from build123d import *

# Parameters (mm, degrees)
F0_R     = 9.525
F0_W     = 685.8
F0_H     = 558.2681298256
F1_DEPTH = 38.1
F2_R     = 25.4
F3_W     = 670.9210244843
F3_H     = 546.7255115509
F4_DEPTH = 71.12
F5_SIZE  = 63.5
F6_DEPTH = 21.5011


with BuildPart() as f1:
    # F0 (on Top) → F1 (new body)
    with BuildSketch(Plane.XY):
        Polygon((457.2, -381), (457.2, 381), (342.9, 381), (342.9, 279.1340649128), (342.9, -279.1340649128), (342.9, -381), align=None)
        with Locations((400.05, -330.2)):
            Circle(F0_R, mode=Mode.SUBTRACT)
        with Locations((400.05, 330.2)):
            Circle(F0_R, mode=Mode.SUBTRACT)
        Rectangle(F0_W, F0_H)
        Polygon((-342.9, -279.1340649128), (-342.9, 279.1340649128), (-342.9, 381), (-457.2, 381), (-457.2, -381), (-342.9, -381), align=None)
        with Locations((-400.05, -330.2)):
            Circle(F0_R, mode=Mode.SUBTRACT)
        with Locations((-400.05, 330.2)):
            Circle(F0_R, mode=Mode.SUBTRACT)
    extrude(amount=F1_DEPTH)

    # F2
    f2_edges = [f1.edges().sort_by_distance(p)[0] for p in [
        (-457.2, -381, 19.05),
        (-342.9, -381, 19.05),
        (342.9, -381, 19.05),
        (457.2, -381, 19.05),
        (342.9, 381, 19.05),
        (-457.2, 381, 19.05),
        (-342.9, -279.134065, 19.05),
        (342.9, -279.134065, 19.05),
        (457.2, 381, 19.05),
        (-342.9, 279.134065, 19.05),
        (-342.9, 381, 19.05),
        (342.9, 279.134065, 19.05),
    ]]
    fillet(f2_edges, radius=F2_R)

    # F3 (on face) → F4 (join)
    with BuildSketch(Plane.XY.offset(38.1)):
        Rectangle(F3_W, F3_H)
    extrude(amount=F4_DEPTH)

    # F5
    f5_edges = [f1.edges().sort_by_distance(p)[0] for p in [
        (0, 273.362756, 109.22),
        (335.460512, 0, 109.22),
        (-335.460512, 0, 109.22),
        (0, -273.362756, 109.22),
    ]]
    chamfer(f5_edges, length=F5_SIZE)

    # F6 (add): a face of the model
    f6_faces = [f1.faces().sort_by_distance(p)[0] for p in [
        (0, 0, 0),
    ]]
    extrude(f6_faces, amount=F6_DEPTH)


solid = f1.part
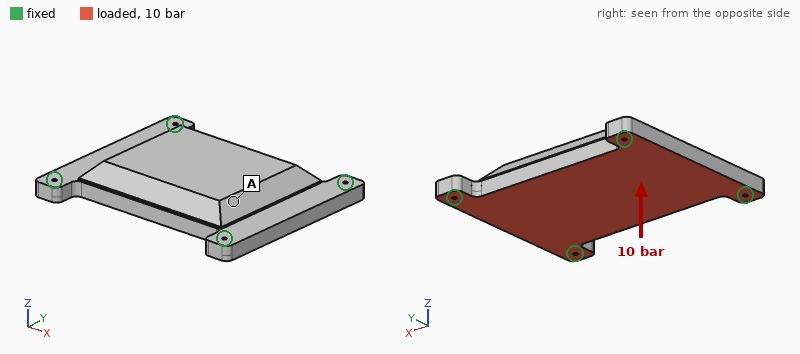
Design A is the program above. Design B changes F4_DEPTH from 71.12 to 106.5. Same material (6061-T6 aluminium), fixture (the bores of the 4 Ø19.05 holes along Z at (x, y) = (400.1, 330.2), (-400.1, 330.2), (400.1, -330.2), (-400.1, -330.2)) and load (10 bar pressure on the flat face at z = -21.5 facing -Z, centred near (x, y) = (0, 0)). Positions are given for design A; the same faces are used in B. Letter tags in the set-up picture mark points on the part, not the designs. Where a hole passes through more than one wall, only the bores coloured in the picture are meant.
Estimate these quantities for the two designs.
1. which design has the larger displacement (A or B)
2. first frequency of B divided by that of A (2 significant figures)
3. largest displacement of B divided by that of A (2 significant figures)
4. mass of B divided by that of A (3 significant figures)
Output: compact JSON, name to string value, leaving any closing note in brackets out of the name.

{"which design has the larger displacement": "A", "first frequency of B divided by that of A": "1.0", "largest displacement of B divided by that of A": "0.72", "mass of B divided by that of A": "1.24"}
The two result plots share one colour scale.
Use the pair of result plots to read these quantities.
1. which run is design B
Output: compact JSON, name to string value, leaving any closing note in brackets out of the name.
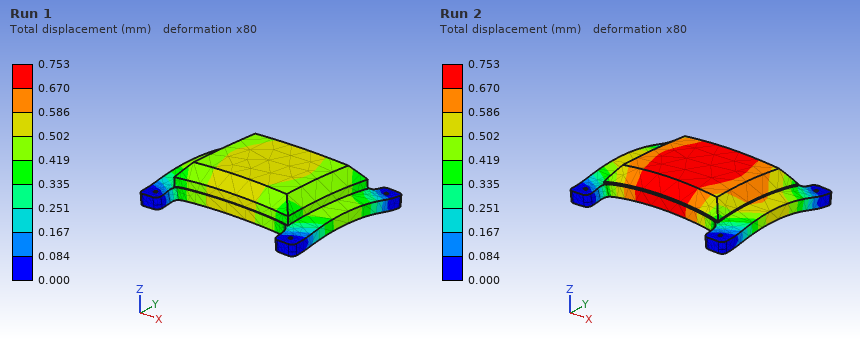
{"which run is design B": "Run 1"}
